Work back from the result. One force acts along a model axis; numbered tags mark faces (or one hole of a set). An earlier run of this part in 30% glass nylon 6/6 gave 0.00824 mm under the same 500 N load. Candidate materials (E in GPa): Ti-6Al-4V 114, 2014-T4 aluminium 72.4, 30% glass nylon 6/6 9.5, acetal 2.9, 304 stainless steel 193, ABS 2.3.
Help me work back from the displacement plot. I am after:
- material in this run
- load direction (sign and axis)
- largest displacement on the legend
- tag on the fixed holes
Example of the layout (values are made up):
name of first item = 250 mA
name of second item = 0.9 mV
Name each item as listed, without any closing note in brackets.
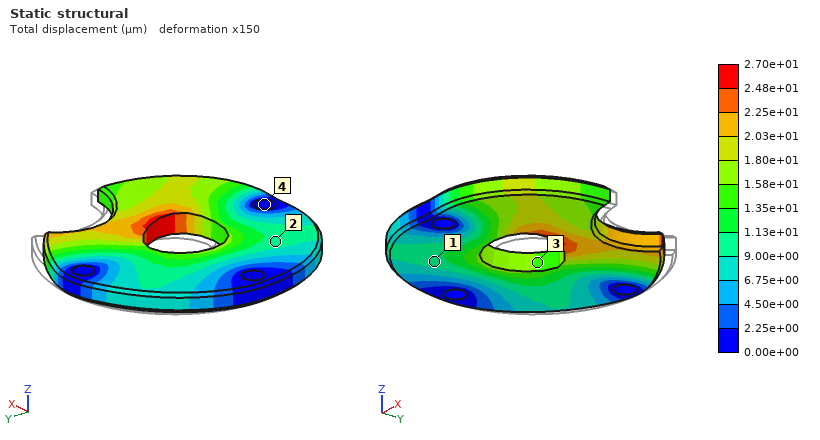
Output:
material in this run = acetal
load direction = -Y
largest displacement on the legend = 2.70e+01 µm
tag on the fixed holes = 4
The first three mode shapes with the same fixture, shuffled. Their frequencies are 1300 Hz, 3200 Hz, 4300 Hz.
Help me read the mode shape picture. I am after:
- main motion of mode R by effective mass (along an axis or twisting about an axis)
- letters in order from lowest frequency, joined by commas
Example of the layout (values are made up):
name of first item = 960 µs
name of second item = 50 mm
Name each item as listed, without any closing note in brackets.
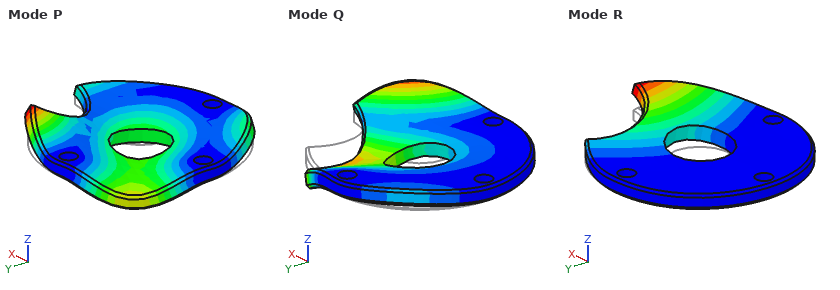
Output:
main motion of mode R by effective mass = along Z
letters in order from lowest frequency, joined by commas = R, Q, P
